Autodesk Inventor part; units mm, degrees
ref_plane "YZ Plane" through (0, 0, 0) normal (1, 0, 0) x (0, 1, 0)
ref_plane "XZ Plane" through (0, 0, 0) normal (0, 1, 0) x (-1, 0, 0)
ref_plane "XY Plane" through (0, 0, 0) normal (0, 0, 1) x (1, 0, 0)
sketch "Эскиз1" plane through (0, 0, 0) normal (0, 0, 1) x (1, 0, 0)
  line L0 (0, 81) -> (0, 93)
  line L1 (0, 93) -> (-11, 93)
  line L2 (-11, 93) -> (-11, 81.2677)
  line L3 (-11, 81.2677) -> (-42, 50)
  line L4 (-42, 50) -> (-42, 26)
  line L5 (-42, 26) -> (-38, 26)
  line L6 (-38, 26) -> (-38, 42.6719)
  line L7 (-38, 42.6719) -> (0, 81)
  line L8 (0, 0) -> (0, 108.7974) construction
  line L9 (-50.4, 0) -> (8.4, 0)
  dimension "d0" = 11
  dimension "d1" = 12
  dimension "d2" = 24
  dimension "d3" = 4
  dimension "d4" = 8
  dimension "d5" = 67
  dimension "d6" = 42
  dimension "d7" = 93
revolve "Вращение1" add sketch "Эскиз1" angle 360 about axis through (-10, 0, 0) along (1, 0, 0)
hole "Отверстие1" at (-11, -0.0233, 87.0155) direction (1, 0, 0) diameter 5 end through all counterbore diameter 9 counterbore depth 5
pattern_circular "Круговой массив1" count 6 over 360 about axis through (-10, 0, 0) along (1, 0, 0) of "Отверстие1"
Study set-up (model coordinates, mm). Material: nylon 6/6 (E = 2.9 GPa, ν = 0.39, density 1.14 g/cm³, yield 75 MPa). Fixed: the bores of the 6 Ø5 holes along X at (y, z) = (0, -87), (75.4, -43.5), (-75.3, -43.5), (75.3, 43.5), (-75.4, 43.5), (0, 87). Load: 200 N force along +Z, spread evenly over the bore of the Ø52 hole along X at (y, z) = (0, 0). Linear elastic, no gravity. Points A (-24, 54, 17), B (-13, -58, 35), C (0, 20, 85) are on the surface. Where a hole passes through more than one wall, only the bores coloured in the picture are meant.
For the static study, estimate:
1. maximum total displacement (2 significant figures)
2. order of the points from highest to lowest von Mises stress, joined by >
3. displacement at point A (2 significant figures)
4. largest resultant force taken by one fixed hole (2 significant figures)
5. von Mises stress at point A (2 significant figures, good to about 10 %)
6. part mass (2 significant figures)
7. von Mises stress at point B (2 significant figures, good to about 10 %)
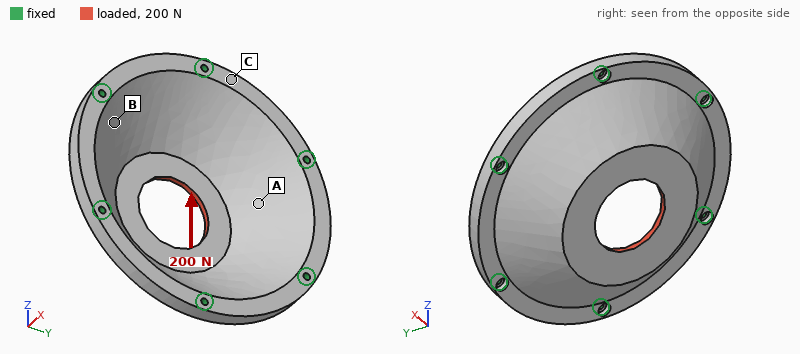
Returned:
22 µm
A > B > C
4.2 µm
44 N
0.26 MPa
280 g
0.13 MPa
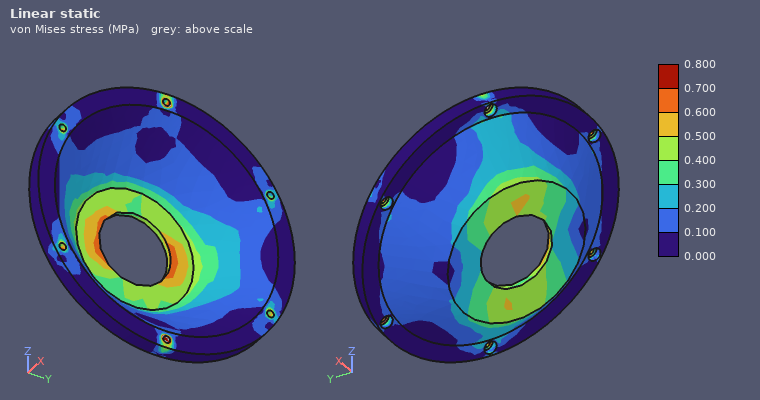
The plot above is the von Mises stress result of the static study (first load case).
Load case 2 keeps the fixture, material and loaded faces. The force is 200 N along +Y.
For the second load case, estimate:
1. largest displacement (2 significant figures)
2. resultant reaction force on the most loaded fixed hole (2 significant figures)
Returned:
22 µm
41 N
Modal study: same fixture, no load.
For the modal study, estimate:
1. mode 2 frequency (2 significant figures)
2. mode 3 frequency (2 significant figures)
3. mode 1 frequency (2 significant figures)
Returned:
2000 Hz
2000 Hz
1900 Hz
